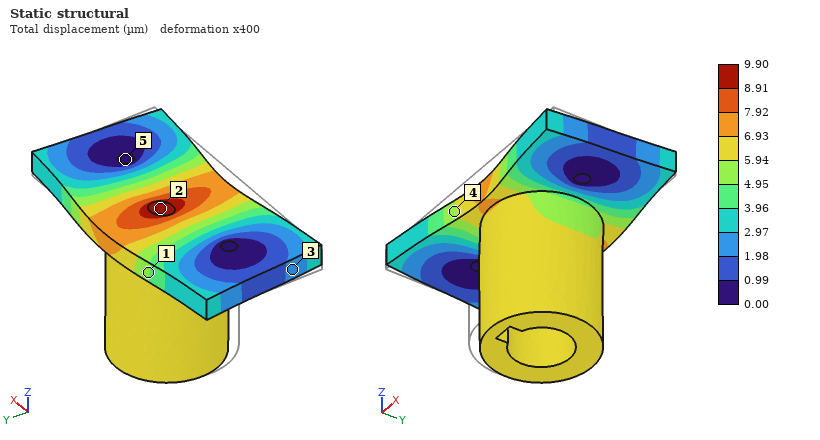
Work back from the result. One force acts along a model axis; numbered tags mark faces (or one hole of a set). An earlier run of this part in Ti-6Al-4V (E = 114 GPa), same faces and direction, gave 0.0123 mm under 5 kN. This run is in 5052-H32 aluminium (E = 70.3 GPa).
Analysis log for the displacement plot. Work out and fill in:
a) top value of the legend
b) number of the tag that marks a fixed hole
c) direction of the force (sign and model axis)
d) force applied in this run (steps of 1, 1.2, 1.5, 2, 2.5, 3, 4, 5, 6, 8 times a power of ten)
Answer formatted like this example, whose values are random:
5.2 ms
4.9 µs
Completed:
9.90 µm
5
+Y
2.5 kN
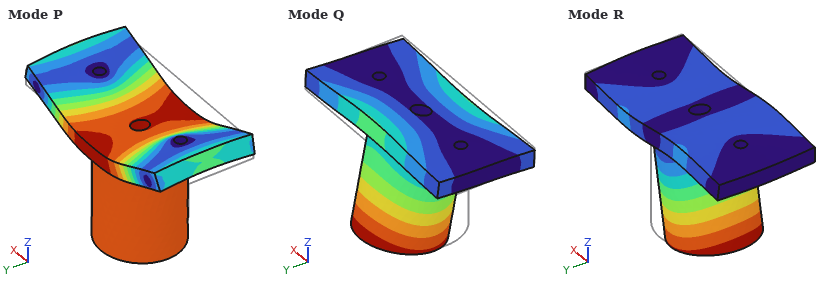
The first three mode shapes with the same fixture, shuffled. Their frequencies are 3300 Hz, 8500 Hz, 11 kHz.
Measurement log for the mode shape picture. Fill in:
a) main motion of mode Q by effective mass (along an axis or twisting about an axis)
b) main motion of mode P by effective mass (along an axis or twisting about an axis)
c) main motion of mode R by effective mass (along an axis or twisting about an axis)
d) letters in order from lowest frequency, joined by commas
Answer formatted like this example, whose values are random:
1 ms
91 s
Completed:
along Y
along Z
along X
Q, R, P
